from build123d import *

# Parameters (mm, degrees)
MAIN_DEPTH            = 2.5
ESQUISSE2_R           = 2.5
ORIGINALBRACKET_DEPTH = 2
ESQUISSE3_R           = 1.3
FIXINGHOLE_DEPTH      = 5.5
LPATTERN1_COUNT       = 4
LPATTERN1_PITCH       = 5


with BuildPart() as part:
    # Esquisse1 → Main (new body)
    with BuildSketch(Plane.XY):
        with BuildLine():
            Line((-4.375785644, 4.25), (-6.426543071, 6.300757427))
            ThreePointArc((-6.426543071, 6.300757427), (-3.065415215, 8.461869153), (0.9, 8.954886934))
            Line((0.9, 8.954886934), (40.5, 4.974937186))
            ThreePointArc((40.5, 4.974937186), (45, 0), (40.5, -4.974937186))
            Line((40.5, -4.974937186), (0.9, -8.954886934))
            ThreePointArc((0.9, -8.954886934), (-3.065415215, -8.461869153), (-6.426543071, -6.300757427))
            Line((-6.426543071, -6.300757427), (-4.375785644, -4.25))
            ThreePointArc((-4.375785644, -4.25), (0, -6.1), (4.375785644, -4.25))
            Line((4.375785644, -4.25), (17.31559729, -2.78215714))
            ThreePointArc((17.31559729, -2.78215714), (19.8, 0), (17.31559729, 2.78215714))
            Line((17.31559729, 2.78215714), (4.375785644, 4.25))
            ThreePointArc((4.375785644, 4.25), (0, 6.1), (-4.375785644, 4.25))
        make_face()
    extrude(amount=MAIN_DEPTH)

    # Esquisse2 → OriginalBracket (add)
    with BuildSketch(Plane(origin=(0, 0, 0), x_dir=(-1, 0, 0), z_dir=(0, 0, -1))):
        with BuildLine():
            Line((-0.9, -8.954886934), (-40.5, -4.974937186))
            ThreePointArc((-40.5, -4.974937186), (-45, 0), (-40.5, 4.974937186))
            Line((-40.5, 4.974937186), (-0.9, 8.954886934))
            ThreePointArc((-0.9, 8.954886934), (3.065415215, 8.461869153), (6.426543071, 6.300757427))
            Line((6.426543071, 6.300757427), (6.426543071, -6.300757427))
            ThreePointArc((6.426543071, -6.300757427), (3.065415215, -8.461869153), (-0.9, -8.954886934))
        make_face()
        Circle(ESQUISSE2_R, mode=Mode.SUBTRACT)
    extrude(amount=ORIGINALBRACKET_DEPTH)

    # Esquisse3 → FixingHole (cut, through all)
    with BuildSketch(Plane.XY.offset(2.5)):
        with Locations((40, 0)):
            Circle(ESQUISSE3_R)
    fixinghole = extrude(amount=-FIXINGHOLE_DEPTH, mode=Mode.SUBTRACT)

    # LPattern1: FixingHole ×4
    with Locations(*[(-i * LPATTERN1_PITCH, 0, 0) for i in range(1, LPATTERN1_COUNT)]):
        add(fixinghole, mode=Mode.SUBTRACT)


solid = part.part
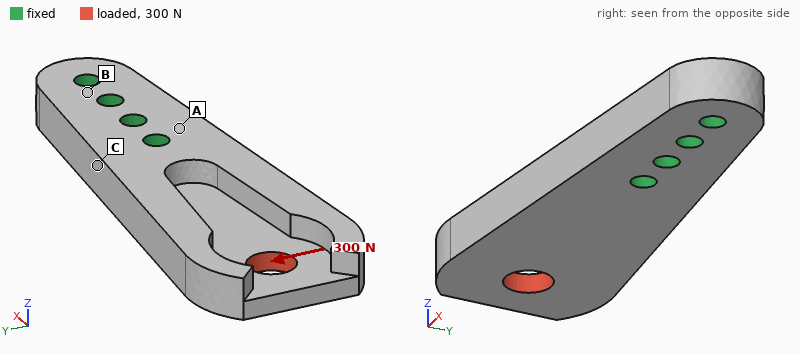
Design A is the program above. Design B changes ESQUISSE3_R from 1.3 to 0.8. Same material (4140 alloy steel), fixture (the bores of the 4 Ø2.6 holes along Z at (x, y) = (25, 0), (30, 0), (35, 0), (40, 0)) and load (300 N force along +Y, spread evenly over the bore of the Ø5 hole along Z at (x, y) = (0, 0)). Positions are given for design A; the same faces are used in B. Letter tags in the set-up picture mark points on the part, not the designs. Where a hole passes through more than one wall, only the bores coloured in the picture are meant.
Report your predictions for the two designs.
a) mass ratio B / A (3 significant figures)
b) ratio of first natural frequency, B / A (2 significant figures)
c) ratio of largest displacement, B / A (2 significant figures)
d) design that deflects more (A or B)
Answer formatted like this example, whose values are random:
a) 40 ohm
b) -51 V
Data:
a) 1.02
b) 0.96
c) 1.1
d) B
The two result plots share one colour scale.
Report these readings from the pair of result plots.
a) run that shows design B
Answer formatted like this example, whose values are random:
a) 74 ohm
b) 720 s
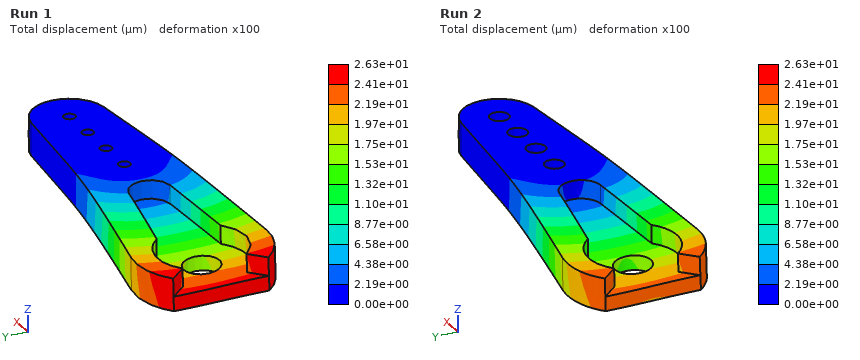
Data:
a) Run 1
